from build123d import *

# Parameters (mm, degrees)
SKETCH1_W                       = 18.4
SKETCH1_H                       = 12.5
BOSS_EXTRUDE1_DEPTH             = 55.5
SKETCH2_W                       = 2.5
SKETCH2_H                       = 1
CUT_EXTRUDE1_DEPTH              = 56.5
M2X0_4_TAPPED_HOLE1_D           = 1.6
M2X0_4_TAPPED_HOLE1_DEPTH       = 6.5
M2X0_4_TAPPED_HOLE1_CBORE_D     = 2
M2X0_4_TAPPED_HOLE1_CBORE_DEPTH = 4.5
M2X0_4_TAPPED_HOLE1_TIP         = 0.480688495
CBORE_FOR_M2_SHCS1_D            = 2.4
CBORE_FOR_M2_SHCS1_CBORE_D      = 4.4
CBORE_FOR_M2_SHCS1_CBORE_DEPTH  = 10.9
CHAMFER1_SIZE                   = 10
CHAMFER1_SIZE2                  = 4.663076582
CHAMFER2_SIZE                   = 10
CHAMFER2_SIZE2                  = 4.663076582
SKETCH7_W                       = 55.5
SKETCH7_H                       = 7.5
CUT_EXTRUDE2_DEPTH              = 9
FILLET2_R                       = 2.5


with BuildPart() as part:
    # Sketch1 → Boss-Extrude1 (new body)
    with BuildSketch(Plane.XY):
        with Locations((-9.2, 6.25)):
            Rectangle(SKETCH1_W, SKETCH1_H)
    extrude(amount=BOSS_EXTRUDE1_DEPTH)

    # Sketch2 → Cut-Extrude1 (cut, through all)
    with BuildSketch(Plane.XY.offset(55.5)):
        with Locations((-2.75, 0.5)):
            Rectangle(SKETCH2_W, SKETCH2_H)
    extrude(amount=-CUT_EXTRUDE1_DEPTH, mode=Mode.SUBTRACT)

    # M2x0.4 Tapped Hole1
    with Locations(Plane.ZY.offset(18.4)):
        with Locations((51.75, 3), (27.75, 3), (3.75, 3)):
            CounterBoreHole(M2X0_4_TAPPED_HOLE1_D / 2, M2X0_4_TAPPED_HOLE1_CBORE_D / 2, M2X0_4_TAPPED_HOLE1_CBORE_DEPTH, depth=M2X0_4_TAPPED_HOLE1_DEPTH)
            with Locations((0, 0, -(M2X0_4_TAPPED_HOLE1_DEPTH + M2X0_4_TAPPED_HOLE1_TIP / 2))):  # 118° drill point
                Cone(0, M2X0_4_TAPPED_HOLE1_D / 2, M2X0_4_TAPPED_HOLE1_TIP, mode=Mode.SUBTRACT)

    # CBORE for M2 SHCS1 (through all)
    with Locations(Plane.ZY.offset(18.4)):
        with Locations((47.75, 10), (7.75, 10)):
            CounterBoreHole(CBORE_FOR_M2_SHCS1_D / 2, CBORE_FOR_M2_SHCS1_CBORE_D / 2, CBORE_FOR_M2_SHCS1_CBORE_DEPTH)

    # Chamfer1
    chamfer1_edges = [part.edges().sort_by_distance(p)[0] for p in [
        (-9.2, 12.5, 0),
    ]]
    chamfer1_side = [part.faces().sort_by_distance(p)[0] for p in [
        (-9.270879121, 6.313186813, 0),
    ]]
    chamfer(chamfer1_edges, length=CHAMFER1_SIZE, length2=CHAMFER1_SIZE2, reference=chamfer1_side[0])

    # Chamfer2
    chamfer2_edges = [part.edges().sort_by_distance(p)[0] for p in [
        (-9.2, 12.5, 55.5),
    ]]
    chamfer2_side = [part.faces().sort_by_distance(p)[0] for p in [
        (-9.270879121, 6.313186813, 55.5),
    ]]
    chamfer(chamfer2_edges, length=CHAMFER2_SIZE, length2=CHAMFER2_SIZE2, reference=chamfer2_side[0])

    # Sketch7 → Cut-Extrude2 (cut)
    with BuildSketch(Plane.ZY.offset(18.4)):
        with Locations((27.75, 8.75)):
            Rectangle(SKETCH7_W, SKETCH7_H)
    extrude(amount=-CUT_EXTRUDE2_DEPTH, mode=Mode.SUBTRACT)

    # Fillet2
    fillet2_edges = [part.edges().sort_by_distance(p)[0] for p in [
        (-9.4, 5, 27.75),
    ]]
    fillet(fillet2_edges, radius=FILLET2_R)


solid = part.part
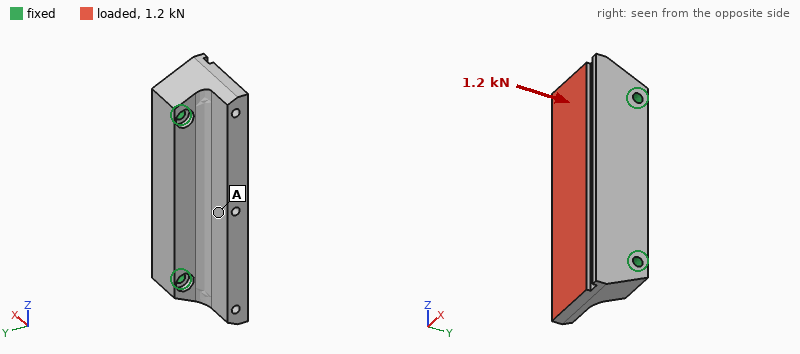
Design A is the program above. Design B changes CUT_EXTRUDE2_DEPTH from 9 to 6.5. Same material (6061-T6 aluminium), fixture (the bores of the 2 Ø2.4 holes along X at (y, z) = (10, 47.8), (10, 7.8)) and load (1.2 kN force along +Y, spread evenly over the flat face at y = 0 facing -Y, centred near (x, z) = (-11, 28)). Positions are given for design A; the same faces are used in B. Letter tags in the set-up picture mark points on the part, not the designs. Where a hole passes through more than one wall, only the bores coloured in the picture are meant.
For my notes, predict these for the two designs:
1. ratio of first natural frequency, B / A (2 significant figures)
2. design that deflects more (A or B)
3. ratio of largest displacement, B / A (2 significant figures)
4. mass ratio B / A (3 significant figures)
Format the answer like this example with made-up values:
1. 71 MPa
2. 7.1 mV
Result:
1. 1.0
2. A
3. 0.83
4. 1.10
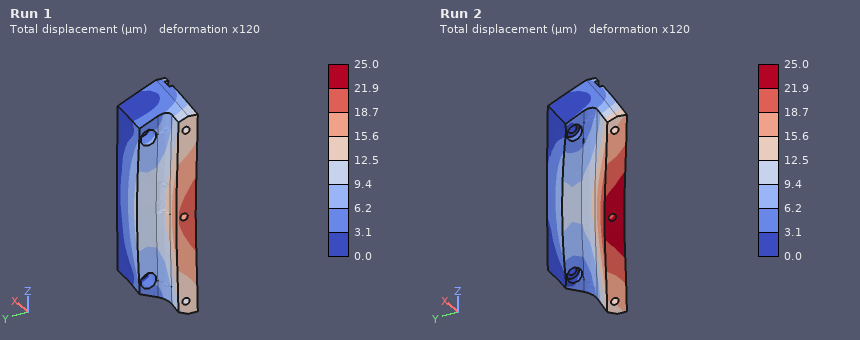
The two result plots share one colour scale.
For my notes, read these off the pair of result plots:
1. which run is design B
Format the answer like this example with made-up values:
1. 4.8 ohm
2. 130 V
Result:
1. Run 1
